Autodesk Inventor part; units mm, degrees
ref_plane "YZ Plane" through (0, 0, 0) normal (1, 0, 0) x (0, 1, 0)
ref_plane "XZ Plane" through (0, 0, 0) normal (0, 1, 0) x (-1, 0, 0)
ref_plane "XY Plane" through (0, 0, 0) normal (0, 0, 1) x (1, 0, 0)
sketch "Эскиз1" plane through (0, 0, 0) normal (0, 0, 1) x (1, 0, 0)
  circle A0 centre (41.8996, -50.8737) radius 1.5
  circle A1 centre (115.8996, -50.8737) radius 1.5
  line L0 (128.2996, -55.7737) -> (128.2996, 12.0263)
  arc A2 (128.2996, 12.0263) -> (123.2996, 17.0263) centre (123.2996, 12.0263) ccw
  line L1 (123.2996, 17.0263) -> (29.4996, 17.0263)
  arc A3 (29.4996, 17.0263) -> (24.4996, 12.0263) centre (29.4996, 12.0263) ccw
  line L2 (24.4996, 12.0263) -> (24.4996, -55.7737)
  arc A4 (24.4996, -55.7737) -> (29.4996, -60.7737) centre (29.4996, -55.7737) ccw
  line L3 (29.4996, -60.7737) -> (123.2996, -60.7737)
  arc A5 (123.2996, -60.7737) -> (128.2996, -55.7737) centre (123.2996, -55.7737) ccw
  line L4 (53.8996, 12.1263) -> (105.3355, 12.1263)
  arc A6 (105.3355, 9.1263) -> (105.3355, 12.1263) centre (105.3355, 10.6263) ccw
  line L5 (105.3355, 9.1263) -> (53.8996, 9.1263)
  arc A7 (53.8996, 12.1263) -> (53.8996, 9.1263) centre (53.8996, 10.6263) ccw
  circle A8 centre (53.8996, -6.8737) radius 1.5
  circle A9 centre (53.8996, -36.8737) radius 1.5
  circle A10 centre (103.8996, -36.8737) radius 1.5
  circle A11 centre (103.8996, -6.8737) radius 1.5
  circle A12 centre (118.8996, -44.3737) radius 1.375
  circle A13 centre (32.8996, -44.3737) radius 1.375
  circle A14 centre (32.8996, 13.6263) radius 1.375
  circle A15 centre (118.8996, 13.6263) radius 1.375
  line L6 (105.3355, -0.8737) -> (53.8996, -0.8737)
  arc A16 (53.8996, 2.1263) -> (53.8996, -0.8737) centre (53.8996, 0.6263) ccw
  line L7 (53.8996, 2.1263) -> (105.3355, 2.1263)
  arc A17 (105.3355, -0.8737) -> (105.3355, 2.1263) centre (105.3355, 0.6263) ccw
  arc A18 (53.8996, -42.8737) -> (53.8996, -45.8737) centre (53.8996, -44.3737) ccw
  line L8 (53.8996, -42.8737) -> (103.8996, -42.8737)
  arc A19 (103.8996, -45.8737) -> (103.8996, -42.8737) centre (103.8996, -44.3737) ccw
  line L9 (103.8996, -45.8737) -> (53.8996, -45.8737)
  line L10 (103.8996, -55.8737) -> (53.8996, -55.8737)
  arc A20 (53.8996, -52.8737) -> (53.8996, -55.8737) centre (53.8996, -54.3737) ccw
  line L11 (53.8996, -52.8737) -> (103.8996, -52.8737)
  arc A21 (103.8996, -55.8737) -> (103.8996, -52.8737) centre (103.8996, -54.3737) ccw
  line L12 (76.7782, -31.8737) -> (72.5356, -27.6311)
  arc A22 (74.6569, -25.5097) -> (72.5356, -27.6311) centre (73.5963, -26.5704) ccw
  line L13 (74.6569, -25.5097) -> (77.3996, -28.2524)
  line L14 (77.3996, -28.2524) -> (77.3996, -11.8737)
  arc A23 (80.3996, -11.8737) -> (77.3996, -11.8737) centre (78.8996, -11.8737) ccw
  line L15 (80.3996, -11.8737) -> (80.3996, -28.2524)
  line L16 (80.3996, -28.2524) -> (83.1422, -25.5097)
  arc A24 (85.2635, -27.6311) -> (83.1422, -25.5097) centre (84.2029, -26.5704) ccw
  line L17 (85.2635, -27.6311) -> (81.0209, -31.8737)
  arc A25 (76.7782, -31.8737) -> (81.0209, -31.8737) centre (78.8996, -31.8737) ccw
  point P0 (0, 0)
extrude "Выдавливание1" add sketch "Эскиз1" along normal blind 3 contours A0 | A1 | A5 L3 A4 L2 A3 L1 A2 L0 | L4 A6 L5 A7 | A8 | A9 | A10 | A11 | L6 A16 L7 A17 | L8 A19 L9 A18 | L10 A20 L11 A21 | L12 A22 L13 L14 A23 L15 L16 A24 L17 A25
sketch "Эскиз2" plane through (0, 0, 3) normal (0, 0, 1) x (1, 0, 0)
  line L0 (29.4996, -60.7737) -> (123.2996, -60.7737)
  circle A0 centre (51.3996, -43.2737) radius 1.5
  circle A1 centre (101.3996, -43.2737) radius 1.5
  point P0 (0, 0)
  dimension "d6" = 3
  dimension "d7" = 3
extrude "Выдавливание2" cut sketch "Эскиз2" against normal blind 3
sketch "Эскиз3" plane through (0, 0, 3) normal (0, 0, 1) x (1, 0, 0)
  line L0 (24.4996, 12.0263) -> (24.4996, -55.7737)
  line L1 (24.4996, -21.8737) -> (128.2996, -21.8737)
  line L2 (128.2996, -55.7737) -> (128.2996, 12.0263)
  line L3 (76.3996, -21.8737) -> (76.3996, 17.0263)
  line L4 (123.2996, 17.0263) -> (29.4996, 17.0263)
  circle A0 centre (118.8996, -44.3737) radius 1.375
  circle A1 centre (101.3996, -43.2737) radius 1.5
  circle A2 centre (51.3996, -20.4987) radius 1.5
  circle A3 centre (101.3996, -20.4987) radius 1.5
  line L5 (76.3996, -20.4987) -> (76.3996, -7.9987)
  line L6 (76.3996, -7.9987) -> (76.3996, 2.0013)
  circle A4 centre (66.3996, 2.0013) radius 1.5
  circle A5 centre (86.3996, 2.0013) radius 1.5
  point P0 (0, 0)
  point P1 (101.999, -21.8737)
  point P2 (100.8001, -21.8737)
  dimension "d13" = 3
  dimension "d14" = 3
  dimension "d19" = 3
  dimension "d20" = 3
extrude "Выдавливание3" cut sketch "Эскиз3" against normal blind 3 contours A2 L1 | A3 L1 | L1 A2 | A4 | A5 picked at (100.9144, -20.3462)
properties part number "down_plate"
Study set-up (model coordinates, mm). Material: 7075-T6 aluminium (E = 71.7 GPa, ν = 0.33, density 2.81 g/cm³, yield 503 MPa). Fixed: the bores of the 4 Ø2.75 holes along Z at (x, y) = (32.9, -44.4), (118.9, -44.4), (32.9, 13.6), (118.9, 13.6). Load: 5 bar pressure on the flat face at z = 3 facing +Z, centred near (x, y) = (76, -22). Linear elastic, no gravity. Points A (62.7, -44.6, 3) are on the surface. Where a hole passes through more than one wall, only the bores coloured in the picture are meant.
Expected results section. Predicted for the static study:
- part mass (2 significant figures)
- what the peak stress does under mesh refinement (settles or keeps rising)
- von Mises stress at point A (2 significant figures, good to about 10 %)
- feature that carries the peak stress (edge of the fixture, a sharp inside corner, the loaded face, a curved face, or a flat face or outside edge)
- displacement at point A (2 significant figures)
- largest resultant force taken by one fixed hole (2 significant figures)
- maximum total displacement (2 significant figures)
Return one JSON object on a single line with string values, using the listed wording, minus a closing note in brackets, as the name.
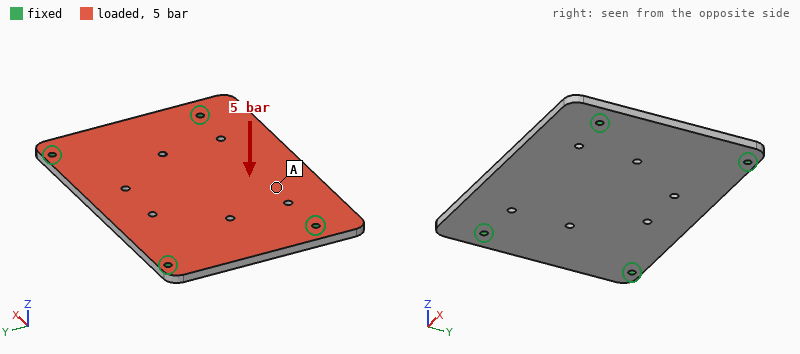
{"part mass": "67 g", "what the peak stress does under mesh refinement": "keeps rising", "von Mises stress at point A": "98 MPa", "feature that carries the peak stress": "edge of the fixture", "displacement at point A": "0.55 mm", "largest resultant force taken by one fixed hole": "1.2 kN", "maximum total displacement": "0.72 mm"}
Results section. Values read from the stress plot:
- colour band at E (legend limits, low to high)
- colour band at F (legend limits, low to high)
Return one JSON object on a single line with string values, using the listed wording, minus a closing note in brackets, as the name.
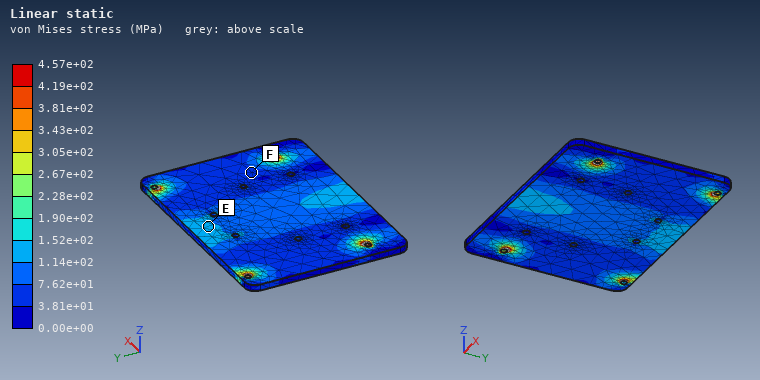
{"colour band at E": "1.14e+02 to 1.52e+02 MPa", "colour band at F": "3.81e+01 to 7.62e+01 MPa"}
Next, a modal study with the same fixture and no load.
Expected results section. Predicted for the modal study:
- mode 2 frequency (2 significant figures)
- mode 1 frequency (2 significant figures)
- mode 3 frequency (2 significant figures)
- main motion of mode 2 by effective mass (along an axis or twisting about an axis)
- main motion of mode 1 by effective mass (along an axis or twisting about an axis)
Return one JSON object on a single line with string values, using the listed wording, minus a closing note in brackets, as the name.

{"mode 2 frequency": "2300 Hz", "mode 1 frequency": "1700 Hz", "mode 3 frequency": "3700 Hz", "main motion of mode 2 by effective mass": "twisting about X", "main motion of mode 1 by effective mass": "along Z"}
